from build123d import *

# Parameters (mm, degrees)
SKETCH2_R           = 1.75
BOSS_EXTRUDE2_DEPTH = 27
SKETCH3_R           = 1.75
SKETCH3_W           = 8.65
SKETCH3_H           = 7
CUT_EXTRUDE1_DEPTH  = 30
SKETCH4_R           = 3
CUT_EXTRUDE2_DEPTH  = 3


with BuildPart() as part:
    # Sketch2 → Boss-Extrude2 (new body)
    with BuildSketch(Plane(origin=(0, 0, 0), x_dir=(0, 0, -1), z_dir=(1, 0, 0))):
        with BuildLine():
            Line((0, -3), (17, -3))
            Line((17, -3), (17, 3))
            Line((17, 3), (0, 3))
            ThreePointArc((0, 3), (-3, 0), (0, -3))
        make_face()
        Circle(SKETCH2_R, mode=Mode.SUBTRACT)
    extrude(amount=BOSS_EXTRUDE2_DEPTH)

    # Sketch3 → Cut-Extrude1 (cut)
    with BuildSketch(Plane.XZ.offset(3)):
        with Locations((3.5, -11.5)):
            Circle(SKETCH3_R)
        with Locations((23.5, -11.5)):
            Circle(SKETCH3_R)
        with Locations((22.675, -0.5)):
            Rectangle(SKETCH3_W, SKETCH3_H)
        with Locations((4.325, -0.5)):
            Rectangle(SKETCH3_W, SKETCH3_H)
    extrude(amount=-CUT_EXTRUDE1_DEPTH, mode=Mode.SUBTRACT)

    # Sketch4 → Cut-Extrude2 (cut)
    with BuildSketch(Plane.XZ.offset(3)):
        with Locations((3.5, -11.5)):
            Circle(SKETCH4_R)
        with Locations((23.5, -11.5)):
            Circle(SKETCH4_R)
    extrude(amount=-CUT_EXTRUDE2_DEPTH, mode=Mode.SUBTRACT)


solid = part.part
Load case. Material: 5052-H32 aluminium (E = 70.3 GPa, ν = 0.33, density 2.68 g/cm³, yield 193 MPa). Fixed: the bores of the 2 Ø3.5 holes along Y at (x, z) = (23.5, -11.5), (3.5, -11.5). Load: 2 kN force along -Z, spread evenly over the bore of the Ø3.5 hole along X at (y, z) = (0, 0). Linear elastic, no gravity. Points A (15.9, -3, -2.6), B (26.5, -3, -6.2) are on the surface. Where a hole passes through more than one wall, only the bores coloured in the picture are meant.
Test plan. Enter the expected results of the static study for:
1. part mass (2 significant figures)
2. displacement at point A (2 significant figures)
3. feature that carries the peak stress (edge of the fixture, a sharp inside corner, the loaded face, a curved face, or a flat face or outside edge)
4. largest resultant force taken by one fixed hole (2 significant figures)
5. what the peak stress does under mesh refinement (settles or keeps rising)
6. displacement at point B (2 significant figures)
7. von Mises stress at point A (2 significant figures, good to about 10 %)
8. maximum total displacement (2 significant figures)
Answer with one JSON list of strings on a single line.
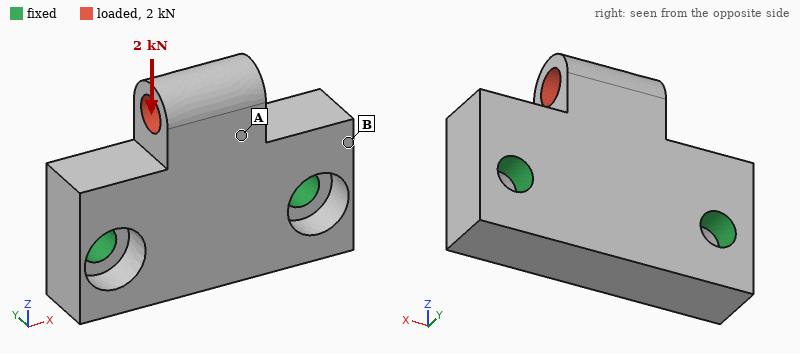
["5.8 g", "17 µm", "edge of the fixture", "1.0 kN", "keeps rising", "5.0 µm", "51 MPa", "23 µm"]
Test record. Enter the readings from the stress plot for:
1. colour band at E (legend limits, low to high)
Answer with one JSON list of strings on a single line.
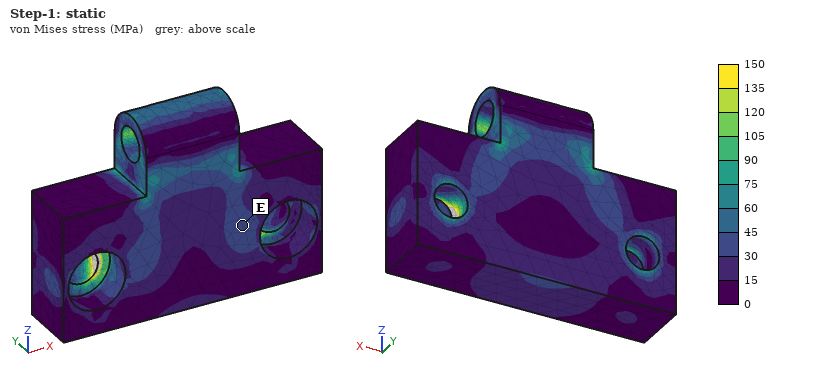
["30 to 45 MPa"]
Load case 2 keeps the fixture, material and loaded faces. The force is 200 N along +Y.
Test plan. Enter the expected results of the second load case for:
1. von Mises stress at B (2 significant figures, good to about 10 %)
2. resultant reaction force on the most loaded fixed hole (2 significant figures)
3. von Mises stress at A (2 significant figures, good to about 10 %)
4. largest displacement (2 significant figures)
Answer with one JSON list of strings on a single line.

["5.9 MPa", "120 N", "18 MPa", "22 µm"]
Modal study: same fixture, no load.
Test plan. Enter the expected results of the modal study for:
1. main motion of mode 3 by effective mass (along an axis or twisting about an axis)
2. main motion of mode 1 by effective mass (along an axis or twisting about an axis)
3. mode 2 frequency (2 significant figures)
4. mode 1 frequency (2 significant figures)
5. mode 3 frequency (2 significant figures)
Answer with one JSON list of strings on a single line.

["along Z", "along Y", "41 kHz", "18 kHz", "49 kHz"]
